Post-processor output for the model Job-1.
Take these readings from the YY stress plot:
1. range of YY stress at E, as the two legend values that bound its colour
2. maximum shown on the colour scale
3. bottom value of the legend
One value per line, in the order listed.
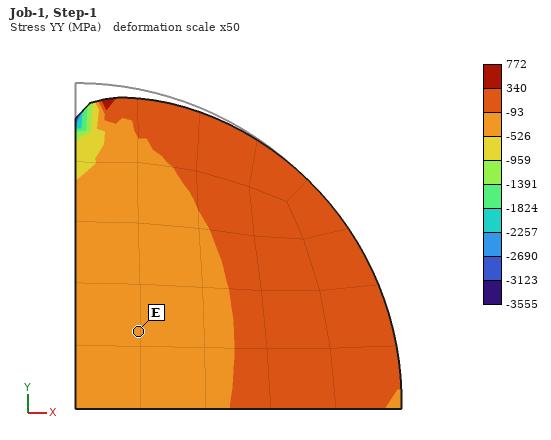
-526 to -93 MPa
772 MPa
-3555 MPa
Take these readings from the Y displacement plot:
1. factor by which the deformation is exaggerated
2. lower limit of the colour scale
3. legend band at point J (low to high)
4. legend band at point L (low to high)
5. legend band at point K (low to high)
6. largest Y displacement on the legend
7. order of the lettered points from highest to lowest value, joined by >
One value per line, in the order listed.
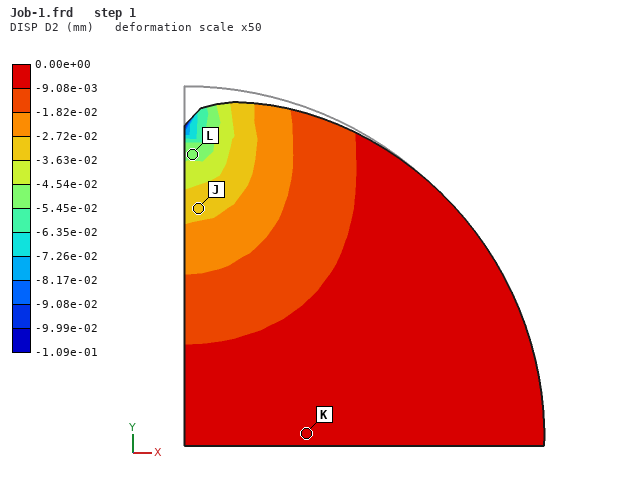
50
-1.09e-01 mm
-3.63e-02 to -2.72e-02 mm
-5.45e-02 to -4.54e-02 mm
-9.08e-03 to 0.00e+00 mm
0.00e+00 mm
K > J > L
